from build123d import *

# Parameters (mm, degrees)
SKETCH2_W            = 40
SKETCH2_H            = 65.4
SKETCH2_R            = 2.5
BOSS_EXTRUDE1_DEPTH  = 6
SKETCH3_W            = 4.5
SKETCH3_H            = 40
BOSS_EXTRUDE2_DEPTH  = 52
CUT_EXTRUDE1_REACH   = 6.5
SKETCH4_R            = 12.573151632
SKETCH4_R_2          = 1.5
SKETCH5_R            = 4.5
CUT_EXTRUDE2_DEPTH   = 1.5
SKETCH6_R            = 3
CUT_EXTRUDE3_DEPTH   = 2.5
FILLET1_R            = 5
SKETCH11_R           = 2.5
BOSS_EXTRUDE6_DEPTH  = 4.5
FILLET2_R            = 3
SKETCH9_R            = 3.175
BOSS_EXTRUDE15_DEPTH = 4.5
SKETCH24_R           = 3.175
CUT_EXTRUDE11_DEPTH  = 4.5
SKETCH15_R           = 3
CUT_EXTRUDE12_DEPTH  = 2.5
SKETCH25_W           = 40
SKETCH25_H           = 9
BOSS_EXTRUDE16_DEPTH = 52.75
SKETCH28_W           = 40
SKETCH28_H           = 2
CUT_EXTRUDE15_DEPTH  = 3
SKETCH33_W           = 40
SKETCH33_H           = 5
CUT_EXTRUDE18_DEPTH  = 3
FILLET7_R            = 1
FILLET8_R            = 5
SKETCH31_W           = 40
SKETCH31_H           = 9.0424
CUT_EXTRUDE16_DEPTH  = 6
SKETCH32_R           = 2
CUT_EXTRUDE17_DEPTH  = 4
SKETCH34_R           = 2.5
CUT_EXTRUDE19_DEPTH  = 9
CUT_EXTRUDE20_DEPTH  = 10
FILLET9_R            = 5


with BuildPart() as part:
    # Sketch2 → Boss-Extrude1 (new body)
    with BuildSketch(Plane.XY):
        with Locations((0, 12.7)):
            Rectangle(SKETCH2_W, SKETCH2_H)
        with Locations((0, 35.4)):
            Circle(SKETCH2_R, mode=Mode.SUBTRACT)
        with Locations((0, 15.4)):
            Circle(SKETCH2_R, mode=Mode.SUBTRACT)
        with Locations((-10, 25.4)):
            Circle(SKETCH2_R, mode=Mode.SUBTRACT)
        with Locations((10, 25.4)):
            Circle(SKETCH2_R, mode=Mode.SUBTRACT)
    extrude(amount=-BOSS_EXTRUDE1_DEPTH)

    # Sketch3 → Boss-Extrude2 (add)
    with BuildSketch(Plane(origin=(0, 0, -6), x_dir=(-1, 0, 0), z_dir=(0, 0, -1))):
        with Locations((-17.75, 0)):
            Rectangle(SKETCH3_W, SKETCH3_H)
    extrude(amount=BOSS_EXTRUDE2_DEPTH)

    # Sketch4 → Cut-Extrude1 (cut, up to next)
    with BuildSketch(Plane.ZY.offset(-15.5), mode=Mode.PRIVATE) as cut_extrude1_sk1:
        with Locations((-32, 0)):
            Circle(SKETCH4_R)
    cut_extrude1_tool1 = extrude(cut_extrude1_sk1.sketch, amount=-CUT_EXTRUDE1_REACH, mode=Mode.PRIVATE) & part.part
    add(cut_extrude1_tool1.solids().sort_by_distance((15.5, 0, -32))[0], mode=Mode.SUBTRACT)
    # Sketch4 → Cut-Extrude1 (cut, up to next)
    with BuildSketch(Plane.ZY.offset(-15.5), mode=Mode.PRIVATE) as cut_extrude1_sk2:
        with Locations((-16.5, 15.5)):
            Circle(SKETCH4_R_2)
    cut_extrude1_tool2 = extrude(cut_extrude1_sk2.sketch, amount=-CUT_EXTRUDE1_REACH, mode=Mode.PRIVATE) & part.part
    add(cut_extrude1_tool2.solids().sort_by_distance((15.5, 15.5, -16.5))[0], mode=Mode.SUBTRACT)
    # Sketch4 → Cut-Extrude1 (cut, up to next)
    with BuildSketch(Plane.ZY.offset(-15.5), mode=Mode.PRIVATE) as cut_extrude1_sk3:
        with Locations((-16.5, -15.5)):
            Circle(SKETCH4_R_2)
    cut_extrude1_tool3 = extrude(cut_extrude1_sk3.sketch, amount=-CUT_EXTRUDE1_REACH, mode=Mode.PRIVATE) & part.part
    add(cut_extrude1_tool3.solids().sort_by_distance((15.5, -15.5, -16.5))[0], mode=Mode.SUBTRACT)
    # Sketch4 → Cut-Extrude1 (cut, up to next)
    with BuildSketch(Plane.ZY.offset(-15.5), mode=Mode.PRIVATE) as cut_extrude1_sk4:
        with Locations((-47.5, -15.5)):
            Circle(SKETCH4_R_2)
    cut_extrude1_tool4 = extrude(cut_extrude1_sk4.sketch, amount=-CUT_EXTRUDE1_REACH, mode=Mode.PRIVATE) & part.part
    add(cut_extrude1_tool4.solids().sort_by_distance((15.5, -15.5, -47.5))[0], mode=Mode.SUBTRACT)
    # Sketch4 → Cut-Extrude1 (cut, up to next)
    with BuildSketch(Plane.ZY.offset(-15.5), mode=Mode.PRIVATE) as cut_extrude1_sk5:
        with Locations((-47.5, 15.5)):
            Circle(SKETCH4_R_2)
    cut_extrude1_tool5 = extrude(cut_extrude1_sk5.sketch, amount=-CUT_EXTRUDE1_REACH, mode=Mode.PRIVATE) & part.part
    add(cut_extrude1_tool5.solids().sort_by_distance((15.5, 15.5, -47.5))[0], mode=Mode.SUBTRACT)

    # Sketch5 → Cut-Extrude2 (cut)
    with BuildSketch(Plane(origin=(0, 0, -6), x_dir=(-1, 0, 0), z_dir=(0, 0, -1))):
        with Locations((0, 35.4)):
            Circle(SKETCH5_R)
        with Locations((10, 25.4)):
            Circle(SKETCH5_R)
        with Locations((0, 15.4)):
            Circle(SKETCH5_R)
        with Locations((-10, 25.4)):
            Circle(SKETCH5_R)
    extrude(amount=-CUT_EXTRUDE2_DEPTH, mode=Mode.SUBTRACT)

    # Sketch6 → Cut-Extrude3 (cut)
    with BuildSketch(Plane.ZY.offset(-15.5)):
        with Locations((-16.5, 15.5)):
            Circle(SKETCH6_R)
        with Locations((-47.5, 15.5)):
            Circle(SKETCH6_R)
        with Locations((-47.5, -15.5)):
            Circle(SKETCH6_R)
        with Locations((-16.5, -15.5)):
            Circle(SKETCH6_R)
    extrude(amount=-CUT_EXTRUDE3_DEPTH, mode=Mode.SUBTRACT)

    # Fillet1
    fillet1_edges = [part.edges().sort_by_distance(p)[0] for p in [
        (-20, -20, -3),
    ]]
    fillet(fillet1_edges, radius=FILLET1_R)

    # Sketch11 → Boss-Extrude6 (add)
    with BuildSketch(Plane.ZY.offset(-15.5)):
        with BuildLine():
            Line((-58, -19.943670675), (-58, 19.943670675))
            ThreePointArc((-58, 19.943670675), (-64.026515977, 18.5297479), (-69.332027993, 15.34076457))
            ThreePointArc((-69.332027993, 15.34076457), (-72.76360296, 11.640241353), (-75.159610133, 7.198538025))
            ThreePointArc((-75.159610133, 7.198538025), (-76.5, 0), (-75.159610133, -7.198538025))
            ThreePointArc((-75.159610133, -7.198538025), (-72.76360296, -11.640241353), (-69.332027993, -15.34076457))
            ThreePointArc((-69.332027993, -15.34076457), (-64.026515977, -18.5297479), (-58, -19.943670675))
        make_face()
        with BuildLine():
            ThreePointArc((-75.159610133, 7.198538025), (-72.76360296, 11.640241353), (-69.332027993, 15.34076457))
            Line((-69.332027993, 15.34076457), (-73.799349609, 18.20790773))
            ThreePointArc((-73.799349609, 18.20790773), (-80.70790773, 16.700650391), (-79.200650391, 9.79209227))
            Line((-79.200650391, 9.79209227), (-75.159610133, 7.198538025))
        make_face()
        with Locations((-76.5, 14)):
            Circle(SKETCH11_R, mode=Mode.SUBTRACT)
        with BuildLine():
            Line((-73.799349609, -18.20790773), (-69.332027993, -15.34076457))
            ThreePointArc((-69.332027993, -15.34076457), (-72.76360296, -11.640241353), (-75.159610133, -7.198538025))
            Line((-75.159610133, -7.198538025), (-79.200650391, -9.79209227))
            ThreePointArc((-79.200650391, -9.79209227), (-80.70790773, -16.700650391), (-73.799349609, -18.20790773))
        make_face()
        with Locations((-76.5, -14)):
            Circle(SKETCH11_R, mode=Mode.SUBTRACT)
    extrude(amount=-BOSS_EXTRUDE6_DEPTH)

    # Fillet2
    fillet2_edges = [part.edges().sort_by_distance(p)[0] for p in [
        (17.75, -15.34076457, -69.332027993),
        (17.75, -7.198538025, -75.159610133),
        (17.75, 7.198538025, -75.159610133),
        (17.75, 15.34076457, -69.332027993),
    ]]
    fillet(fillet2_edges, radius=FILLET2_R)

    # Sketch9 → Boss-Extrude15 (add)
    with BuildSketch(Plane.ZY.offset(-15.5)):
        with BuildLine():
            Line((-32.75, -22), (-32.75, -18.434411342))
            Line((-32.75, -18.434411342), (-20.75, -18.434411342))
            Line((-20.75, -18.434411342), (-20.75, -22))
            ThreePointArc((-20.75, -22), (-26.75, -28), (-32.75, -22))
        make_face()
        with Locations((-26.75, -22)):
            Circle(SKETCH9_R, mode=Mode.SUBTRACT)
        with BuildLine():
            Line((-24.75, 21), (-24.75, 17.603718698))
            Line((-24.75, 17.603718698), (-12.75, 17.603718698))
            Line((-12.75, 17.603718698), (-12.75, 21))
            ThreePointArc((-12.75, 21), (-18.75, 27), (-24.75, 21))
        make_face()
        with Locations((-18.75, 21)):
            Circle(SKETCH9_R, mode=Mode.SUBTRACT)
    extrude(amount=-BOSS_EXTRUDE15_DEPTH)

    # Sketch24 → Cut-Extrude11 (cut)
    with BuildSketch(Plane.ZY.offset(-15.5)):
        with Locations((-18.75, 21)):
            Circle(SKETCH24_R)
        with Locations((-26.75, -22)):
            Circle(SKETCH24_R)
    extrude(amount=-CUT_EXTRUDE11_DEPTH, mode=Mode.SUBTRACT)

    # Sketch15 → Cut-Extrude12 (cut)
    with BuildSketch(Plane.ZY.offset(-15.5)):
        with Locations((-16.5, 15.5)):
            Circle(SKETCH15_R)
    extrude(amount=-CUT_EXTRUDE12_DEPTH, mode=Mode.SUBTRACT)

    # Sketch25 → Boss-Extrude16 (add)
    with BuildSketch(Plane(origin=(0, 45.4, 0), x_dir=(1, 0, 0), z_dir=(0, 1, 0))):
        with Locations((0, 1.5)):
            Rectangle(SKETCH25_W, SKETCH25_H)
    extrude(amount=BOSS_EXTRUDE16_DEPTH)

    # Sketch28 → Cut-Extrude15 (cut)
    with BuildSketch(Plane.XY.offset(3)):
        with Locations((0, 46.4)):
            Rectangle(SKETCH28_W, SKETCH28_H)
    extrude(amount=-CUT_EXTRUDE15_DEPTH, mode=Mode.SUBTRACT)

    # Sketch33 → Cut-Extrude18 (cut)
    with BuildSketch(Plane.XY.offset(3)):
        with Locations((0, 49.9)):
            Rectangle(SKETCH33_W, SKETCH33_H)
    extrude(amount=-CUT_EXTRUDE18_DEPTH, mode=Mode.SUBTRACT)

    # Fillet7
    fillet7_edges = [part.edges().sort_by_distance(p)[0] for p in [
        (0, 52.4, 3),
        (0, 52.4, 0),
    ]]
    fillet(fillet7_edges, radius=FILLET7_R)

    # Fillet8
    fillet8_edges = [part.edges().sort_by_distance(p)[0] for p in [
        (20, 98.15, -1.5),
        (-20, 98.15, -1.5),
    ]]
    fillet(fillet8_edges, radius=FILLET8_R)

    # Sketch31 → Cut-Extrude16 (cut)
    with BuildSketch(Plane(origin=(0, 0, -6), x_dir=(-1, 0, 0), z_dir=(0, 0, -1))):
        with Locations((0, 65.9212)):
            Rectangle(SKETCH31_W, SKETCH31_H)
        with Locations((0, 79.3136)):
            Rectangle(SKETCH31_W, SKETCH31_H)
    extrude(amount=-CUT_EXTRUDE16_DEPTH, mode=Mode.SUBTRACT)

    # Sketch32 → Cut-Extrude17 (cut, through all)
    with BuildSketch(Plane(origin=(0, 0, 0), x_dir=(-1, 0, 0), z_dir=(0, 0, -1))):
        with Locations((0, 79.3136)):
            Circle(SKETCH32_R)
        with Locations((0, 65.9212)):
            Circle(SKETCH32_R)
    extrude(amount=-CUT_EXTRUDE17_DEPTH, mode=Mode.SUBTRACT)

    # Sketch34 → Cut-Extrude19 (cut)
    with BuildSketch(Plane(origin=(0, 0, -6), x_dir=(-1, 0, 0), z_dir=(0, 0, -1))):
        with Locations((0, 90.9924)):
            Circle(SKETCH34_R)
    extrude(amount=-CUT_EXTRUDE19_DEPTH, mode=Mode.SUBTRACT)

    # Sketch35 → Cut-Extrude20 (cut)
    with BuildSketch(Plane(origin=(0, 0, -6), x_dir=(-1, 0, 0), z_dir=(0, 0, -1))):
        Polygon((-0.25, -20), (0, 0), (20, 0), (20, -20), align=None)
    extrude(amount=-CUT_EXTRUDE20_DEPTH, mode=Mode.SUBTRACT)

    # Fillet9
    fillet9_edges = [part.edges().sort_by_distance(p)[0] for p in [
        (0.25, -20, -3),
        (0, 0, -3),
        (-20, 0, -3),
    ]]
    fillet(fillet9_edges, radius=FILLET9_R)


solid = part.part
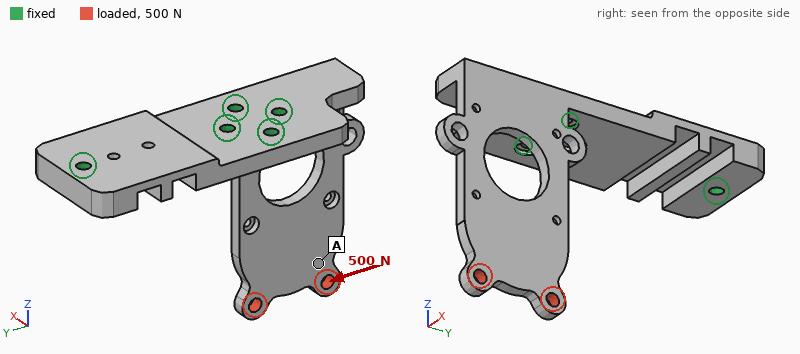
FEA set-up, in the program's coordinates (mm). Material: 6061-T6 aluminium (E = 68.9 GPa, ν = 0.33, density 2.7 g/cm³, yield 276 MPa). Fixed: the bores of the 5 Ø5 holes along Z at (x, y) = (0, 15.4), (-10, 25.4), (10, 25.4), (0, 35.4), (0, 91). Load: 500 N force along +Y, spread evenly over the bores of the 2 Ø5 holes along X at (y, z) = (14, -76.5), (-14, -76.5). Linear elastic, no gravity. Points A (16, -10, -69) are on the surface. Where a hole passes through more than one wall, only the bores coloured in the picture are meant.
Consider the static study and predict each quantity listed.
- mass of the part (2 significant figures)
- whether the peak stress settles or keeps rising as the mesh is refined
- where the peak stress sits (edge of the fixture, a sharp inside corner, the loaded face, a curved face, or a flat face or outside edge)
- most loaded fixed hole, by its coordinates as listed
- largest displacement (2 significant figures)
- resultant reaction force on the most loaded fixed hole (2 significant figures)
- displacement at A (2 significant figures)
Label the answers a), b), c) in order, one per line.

a) 98 g
b) keeps rising
c) edge of the fixture
d) (0, 15.4)
e) 1.2 mm
f) 2.1 kN
g) 0.96 mm
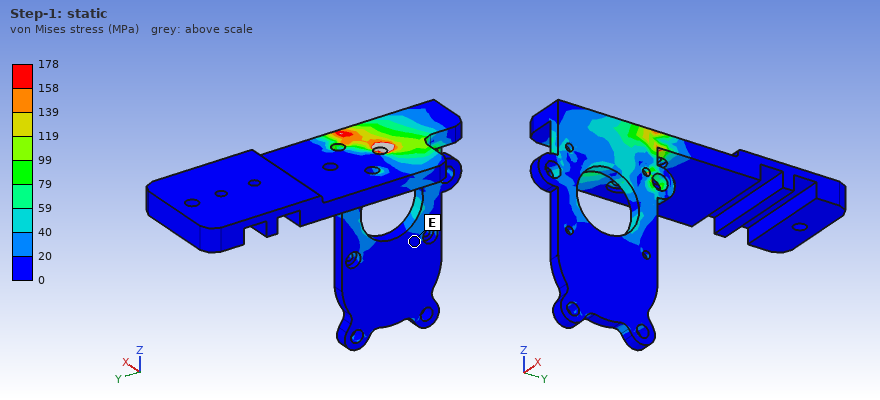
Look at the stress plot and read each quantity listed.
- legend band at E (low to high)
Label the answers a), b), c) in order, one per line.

a) 0 to 20 MPa
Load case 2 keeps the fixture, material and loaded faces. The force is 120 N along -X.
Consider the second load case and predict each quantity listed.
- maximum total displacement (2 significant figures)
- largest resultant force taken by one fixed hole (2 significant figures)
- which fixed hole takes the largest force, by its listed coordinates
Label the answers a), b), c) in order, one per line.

a) 1.7 mm
b) 390 N
c) (10, 25.4)
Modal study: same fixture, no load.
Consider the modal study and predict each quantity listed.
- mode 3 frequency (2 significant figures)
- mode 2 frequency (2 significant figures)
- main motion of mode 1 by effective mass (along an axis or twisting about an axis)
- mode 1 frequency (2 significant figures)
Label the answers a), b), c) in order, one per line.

a) 2100 Hz
b) 1100 Hz
c) along X
d) 490 Hz
